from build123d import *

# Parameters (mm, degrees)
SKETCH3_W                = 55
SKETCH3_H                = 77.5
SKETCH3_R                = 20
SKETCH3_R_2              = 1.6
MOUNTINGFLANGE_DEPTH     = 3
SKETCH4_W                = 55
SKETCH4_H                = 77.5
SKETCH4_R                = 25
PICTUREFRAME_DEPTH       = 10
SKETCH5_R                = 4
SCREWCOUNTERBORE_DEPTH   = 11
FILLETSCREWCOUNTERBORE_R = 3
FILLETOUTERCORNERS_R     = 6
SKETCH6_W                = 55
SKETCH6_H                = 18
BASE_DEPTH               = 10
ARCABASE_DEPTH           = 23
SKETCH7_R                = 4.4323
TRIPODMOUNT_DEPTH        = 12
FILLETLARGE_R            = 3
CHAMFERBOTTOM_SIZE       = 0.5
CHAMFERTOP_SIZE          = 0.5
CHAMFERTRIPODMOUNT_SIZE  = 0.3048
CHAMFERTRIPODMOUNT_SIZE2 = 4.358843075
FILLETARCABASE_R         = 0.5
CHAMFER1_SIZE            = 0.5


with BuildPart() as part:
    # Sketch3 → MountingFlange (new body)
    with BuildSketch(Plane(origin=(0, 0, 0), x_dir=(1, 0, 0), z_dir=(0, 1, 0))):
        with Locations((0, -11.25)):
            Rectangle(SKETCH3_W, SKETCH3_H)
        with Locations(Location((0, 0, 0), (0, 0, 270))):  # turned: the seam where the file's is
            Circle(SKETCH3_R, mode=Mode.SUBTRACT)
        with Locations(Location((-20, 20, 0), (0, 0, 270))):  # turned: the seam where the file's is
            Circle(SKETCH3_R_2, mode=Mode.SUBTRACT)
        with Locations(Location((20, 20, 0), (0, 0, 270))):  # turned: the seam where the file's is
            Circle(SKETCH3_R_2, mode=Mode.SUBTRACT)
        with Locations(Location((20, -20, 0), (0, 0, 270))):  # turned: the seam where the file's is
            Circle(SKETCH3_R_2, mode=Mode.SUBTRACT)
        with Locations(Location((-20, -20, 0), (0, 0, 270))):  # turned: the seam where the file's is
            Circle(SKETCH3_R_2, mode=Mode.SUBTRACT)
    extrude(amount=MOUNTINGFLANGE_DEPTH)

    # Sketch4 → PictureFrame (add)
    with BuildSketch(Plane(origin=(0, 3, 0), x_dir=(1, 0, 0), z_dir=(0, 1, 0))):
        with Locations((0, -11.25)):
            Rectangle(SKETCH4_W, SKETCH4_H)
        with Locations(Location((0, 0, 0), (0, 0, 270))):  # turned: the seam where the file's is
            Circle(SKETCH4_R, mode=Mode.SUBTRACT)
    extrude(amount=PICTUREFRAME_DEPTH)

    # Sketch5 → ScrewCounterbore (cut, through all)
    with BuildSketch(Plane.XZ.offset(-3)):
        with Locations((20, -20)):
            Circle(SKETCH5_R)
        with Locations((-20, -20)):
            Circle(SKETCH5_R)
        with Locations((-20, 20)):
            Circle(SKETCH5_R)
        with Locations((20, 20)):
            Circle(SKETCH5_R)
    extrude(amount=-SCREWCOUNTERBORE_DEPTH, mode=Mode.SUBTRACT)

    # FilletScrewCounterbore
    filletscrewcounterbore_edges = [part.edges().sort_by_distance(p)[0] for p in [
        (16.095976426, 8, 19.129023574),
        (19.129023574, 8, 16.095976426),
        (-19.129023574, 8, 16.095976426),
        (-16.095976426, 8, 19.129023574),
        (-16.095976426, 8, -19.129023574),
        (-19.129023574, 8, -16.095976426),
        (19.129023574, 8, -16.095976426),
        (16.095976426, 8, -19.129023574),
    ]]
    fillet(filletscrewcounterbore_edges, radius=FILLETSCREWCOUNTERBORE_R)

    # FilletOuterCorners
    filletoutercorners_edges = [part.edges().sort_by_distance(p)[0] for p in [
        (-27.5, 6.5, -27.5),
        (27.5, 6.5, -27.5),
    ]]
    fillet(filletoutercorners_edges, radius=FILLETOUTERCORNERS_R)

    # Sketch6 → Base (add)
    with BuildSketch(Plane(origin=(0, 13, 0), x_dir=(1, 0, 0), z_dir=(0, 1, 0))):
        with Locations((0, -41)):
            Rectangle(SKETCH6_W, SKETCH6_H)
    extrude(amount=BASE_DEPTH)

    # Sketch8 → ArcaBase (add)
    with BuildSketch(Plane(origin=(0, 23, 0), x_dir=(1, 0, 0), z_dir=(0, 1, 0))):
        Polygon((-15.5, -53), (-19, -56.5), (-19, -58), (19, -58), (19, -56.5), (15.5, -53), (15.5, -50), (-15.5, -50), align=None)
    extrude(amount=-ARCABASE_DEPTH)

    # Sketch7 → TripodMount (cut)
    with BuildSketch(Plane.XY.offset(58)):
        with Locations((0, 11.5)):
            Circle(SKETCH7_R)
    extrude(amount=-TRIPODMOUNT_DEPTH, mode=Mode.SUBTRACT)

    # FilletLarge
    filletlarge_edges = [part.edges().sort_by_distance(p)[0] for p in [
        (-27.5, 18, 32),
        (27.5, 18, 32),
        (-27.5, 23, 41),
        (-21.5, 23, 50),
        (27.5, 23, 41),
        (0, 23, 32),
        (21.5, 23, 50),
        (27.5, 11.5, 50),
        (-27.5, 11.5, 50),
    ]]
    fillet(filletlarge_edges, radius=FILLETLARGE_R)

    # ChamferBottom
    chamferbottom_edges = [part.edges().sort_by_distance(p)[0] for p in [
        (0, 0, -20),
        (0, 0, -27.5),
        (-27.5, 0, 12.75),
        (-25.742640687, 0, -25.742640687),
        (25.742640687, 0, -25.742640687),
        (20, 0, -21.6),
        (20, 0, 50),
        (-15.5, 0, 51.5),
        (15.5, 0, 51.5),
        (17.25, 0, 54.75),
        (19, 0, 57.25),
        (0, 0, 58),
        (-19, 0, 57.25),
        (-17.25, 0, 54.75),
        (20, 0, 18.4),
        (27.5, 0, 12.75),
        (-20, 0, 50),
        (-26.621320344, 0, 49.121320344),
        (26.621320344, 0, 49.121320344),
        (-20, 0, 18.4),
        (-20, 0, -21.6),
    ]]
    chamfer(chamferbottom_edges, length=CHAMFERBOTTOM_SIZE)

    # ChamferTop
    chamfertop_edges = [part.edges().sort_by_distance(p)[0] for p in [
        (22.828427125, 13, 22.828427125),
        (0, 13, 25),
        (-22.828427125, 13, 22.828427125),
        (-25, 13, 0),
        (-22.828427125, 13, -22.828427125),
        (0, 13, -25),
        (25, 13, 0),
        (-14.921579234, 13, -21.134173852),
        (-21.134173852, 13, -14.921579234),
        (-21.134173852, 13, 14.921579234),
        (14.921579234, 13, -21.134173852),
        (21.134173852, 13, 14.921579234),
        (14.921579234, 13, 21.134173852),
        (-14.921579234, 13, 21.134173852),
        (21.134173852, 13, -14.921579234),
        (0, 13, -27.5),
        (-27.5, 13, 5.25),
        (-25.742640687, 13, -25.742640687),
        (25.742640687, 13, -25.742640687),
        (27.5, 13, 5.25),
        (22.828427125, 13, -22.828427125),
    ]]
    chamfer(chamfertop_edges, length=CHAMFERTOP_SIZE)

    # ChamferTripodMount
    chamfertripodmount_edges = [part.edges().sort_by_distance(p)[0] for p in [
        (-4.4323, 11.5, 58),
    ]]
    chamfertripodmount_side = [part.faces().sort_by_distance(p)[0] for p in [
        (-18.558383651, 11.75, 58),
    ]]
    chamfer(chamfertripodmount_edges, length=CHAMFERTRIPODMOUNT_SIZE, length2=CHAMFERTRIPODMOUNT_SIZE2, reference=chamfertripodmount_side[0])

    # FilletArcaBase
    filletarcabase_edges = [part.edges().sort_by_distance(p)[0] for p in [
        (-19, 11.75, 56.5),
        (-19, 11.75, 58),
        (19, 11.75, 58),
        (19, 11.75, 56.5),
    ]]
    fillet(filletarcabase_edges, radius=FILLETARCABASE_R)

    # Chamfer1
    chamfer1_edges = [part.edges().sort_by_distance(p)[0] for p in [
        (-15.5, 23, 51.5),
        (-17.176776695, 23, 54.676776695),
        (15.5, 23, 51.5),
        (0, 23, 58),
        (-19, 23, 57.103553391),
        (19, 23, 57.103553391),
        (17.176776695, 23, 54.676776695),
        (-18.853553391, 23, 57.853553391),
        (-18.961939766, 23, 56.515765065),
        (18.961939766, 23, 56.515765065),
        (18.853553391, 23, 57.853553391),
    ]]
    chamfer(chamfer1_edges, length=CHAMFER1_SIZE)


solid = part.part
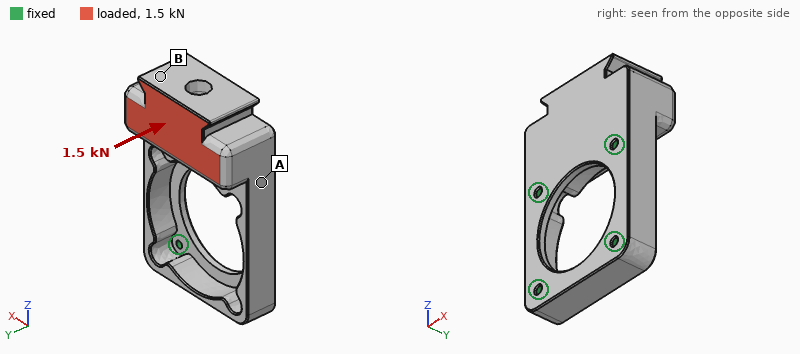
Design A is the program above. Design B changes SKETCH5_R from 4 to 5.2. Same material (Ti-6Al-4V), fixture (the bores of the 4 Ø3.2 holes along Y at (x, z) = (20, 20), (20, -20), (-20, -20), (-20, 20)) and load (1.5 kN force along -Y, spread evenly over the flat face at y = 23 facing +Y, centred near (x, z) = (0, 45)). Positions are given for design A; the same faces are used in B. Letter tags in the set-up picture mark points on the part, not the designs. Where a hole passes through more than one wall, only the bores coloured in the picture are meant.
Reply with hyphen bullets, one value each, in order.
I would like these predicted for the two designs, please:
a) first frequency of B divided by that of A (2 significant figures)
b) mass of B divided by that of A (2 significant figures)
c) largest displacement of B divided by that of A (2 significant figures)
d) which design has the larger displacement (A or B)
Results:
- 0.92
- 0.98
- 1.2
- B
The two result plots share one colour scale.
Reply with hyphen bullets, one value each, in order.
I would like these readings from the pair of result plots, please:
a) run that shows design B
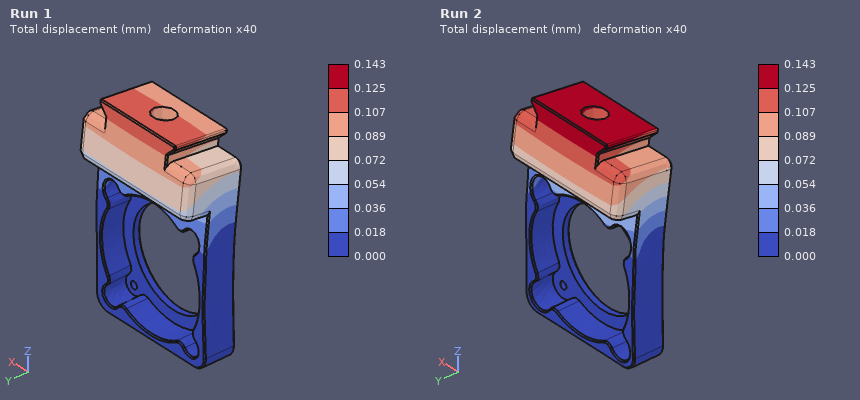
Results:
- Run 2
